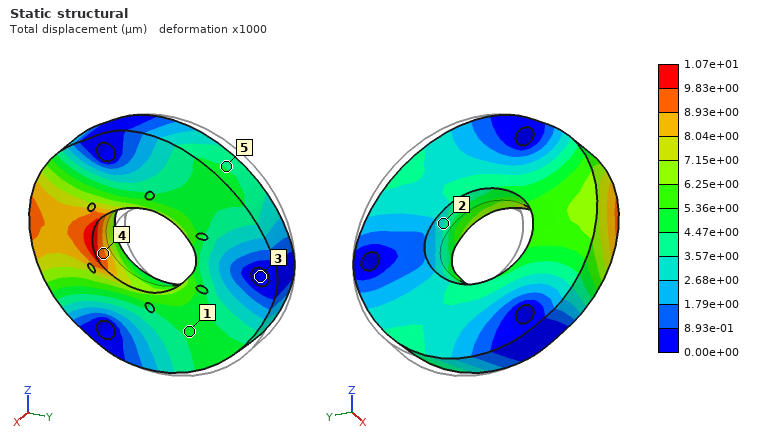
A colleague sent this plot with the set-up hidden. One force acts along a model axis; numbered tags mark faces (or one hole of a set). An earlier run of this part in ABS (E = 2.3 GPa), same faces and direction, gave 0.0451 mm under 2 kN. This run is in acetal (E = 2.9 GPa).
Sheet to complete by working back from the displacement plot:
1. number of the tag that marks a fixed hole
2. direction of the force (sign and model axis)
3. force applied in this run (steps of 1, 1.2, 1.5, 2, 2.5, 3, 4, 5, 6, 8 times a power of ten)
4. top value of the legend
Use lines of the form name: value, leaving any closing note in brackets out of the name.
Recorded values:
number of the tag that marks a fixed hole: 3
direction of the force: -Y
force applied in this run: 600 N
top value of the legend: 1.07e+01 µm
